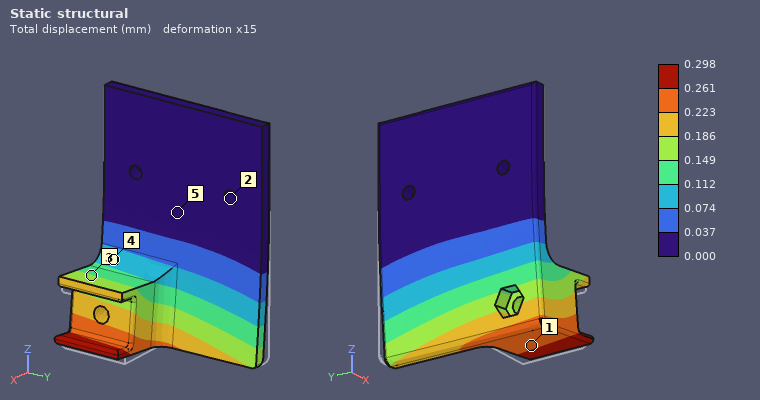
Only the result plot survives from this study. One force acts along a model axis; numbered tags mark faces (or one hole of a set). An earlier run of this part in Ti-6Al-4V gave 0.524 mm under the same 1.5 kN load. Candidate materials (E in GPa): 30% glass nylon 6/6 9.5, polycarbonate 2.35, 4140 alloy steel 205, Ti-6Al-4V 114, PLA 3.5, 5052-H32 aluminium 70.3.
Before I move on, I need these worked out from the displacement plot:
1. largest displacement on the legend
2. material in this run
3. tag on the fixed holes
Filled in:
0.298 mm
4140 alloy steel
2
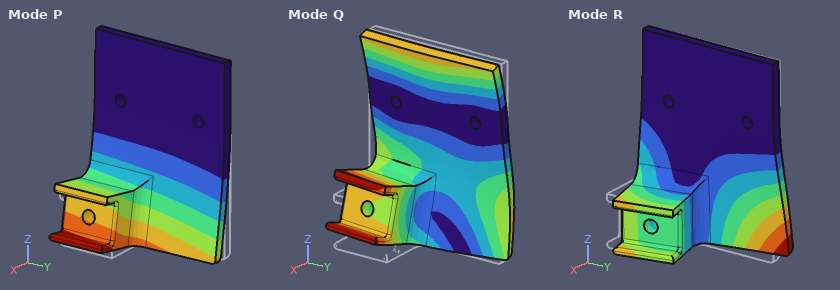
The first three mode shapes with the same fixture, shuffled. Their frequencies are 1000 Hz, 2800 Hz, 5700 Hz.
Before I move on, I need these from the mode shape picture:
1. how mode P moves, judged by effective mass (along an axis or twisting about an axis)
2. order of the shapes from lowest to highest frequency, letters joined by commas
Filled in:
along X
P, R, Q
